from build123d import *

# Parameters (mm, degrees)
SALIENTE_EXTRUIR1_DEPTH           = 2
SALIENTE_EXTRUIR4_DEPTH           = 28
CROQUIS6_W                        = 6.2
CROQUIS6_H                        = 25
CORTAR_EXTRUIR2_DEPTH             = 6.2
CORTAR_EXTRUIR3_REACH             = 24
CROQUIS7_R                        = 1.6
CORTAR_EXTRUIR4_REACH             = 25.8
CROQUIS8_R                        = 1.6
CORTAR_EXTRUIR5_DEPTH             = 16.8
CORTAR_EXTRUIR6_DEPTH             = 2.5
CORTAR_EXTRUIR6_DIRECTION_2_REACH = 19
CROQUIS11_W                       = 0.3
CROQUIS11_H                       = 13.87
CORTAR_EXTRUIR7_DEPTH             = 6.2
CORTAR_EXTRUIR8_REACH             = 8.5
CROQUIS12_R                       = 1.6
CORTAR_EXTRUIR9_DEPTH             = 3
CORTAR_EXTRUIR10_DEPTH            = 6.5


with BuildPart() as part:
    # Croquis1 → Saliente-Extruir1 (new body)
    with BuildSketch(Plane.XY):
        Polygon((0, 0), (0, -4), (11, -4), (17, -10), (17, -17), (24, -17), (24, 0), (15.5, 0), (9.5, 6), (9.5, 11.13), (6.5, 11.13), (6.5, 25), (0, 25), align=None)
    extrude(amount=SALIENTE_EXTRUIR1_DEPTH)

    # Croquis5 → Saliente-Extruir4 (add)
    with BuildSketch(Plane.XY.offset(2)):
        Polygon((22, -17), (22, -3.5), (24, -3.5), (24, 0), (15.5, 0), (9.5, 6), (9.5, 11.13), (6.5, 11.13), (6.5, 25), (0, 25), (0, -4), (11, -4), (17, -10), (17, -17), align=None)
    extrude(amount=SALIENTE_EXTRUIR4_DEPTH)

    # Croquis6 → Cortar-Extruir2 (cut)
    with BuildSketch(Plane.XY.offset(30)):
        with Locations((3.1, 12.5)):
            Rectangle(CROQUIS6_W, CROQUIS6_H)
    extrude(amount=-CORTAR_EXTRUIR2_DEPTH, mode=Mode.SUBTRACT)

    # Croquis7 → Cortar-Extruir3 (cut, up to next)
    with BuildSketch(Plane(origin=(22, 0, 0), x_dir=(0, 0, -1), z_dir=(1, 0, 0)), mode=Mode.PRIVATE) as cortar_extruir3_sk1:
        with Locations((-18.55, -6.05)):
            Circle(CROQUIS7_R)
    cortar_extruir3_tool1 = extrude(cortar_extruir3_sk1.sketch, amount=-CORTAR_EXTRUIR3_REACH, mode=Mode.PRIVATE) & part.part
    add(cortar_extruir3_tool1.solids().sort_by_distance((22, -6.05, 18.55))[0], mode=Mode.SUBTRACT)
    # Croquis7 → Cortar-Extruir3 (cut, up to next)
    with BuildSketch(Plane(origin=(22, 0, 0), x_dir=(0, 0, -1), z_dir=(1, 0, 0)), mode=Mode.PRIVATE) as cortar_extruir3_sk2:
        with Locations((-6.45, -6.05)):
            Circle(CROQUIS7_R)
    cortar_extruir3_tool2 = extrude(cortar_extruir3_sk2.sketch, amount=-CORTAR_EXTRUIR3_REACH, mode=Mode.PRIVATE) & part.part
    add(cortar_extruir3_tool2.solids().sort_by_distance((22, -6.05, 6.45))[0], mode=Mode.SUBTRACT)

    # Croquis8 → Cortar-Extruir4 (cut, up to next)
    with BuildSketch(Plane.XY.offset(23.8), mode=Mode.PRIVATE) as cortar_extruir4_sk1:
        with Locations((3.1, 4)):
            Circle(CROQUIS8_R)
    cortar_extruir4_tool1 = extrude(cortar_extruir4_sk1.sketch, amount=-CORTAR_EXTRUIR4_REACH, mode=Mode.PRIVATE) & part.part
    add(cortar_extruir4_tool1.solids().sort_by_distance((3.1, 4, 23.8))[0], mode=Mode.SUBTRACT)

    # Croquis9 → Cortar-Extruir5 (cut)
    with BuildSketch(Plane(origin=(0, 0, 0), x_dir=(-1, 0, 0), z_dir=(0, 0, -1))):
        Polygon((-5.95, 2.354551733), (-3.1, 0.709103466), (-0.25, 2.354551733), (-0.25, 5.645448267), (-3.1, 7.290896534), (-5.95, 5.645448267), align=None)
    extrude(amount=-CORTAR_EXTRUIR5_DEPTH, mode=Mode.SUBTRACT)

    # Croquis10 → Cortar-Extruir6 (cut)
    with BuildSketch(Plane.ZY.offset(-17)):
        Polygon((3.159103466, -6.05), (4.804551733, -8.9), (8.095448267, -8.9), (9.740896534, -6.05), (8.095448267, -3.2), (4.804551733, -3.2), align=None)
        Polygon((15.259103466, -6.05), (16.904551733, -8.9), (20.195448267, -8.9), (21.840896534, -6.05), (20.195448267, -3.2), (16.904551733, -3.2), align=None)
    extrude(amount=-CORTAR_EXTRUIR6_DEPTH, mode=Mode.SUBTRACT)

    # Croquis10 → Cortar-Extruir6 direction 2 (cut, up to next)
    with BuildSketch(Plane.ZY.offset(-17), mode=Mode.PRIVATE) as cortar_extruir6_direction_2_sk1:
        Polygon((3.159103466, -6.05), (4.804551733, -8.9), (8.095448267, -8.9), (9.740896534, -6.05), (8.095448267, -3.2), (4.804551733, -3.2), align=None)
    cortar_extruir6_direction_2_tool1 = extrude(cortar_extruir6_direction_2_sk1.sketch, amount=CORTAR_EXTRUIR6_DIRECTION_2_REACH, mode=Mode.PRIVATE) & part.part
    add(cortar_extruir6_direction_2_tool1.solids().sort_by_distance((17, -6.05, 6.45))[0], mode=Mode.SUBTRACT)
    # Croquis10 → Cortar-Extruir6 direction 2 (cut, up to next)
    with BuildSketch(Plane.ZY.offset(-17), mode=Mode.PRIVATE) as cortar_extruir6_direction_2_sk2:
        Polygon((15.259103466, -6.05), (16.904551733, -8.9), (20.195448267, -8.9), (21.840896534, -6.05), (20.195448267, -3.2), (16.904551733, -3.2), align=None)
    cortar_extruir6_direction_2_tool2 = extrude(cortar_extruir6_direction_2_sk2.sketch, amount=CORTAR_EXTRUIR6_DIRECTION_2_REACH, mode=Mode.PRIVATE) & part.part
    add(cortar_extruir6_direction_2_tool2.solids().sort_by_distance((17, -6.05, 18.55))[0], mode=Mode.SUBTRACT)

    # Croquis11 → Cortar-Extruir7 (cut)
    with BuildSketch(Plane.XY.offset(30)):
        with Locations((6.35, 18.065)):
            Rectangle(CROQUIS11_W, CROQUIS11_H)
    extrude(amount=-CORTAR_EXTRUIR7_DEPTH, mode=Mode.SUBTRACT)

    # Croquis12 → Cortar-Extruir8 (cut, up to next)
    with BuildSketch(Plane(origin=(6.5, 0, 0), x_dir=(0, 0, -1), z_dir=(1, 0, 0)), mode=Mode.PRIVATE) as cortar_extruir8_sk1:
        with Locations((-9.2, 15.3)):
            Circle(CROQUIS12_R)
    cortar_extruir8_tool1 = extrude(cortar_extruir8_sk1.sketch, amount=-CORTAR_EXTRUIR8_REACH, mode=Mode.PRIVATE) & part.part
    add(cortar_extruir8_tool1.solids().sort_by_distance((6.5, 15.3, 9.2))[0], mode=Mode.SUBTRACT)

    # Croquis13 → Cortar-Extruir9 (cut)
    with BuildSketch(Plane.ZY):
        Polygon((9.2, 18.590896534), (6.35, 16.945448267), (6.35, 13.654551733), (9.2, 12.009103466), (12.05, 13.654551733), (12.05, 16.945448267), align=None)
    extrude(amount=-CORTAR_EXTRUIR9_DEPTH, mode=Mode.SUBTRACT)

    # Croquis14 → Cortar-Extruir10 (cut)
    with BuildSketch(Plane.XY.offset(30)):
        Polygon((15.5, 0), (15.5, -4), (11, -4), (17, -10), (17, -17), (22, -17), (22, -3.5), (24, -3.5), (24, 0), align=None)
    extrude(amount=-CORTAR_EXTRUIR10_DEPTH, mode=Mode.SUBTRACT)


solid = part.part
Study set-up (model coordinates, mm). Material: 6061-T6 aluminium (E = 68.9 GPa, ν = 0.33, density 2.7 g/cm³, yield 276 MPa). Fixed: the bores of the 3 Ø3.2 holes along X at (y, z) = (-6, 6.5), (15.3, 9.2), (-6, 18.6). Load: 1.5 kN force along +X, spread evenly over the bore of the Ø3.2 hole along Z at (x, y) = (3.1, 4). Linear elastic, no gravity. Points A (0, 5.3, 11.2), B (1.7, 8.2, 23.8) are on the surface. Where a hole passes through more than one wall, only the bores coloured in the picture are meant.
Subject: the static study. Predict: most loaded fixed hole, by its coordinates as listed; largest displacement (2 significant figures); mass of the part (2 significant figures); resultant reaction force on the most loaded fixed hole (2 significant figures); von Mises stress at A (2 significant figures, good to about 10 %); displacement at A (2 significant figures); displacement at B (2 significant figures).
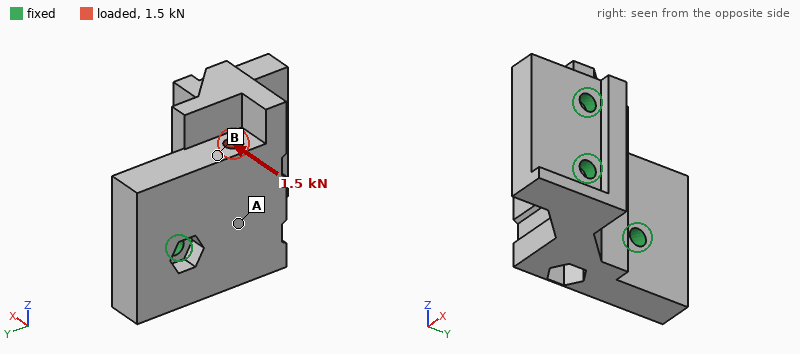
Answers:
(-6, 18.6)
34 µm
24 g
1.2 kN
32 MPa
13 µm
26 µm
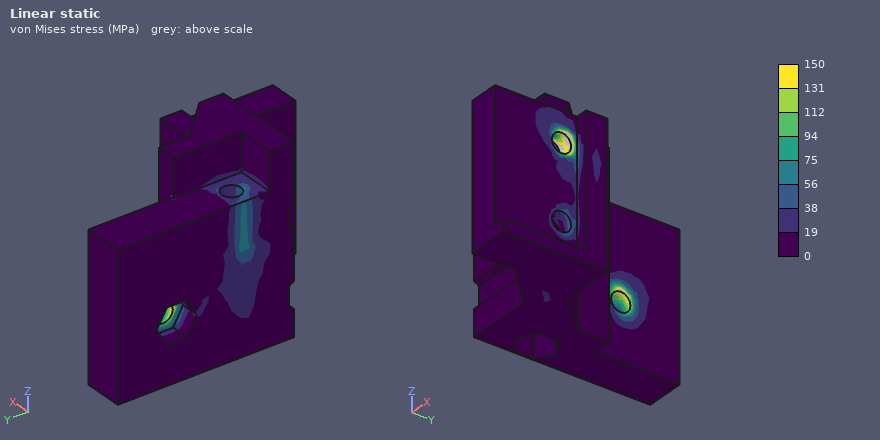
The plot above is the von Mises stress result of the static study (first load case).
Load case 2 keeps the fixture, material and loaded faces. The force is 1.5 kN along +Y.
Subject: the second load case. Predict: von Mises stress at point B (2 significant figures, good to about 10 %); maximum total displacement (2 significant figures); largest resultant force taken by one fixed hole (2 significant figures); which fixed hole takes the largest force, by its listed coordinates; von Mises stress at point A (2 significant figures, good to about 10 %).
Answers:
16 MPa
35 µm
1.4 kN
(15.3, 9.2)
50 MPa
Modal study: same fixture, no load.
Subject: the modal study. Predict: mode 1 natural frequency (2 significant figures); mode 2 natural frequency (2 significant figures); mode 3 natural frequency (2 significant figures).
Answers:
10 kHz
20 kHz
23 kHz
